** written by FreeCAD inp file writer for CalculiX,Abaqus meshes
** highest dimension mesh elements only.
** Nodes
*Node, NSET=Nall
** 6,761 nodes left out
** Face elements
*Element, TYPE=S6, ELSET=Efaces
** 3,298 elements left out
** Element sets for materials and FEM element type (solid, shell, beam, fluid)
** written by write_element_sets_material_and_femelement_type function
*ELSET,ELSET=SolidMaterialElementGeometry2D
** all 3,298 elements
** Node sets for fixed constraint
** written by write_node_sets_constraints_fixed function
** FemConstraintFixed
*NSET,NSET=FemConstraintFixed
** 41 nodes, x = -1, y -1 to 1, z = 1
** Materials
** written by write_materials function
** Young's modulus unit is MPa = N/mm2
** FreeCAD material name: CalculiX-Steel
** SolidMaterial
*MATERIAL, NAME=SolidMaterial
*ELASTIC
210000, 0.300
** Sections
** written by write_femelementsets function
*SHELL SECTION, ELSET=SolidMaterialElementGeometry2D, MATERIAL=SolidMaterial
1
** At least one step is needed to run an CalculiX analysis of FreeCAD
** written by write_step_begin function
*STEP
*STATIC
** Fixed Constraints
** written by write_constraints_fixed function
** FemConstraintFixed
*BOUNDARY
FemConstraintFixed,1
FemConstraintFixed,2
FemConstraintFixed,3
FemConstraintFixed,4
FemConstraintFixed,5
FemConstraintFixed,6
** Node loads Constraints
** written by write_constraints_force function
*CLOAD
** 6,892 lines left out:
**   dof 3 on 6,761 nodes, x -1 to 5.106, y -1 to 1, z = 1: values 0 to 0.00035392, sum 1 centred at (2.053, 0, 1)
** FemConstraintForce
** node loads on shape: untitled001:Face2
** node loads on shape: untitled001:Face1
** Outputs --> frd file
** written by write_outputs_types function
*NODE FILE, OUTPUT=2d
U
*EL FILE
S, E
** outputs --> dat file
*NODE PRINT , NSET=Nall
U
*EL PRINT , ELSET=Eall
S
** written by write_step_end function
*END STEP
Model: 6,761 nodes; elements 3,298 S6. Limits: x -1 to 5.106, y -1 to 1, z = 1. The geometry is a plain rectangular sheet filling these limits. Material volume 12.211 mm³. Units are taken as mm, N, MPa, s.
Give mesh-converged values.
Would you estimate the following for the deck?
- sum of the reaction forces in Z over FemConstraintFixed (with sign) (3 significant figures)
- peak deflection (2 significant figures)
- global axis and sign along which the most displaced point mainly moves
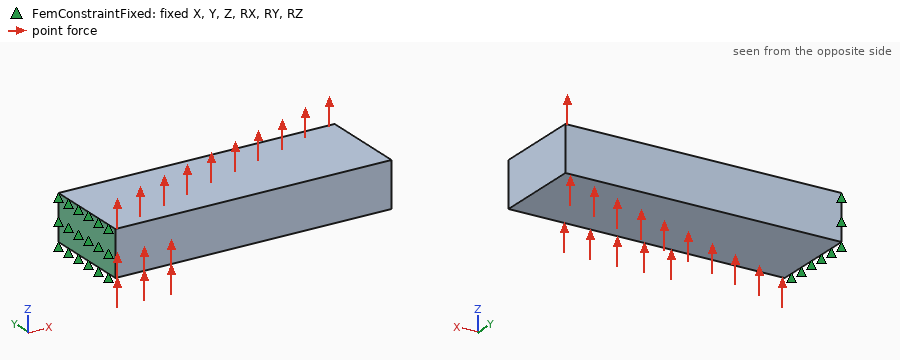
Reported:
-1.00 N
8.1e-04 mm
+Z
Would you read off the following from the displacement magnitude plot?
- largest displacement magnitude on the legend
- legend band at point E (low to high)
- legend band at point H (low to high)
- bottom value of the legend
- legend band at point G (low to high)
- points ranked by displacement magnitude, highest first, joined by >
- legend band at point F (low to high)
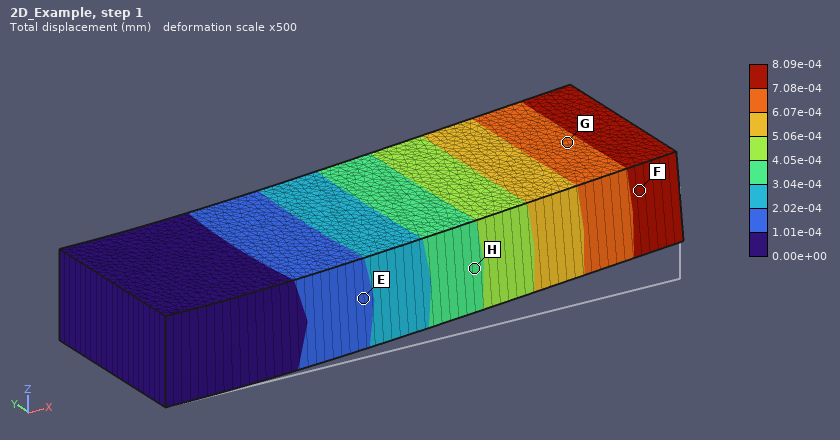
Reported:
8.09e-04 mm
1.01e-04 to 2.02e-04 mm
3.04e-04 to 4.05e-04 mm
0.00e+00 mm
6.07e-04 to 7.08e-04 mm
F > G > H > E
7.08e-04 to 8.09e-04 mm
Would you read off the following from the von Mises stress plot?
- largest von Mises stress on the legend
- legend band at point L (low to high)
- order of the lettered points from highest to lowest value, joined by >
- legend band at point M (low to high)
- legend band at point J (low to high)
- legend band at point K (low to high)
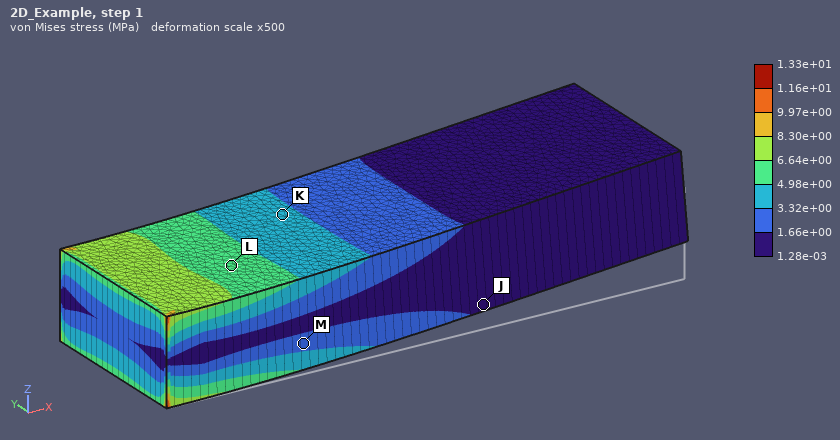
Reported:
1.33e+01 MPa
4.98e+00 to 6.64e+00 MPa
L > K > M > J
1.66e+00 to 3.32e+00 MPa
1.28e-03 to 1.66e+00 MPa
3.32e+00 to 4.98e+00 MPa
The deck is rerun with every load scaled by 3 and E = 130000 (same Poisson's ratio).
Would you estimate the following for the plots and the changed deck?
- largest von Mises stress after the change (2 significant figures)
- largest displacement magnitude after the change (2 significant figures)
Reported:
40 MPa
0.0039 mm
